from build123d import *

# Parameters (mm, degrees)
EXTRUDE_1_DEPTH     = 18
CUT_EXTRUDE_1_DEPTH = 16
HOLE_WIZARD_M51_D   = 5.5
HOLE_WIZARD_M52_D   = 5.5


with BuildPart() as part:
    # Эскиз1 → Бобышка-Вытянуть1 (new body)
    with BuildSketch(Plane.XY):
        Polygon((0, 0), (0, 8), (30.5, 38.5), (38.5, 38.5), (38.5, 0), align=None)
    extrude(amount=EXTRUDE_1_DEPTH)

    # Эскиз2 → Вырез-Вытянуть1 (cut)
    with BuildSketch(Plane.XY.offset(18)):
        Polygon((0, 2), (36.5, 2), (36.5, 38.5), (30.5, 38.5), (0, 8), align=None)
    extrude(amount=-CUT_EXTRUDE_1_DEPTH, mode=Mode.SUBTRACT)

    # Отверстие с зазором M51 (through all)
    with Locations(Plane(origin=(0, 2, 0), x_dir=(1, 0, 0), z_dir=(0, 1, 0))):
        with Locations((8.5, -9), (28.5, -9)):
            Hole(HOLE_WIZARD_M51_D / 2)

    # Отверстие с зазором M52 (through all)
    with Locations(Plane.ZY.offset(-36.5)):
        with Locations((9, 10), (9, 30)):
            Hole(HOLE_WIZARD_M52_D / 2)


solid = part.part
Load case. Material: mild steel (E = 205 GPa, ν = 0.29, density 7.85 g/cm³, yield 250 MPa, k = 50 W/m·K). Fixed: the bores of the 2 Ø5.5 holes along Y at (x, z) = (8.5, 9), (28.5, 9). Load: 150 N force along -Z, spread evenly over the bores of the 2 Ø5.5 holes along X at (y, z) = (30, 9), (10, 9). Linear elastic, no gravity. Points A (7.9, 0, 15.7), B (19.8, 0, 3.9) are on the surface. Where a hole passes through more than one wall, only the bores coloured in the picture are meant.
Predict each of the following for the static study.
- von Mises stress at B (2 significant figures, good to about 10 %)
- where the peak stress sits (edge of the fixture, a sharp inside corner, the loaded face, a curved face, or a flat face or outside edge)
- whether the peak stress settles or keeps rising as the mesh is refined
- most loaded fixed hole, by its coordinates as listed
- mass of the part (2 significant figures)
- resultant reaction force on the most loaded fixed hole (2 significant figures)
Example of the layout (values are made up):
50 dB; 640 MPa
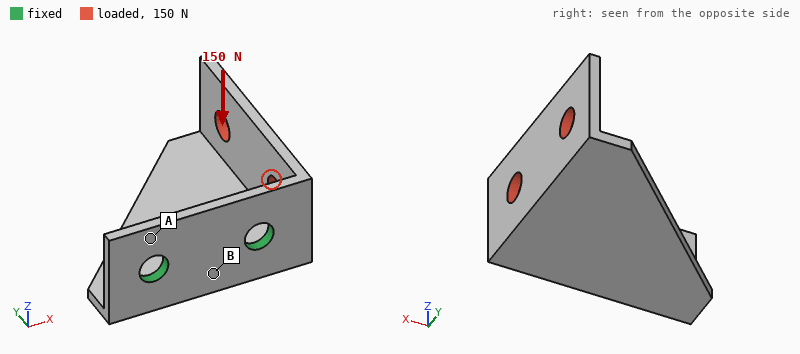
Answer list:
35 MPa; edge of the fixture; keeps rising; (28.5, 9); 33 g; 180 N
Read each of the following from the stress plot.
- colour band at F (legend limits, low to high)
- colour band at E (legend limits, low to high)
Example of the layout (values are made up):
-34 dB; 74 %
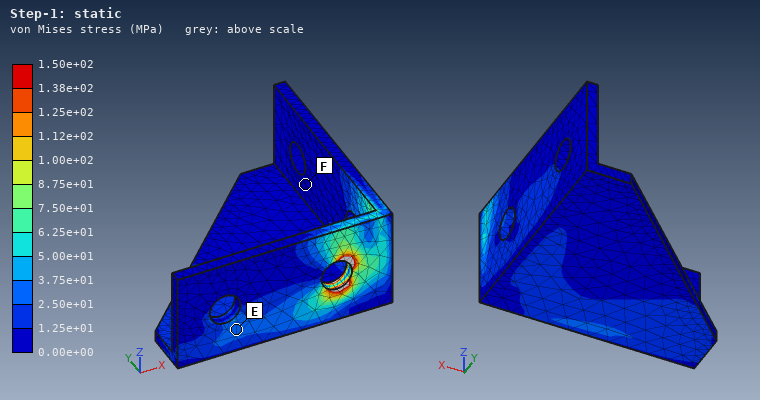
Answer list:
0.00e+00 to 1.25e+01 MPa; 2.50e+01 to 3.75e+01 MPa
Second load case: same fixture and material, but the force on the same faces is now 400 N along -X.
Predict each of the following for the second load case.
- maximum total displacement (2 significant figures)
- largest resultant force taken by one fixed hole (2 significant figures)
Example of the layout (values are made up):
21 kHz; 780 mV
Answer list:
0.16 mm; 390 N
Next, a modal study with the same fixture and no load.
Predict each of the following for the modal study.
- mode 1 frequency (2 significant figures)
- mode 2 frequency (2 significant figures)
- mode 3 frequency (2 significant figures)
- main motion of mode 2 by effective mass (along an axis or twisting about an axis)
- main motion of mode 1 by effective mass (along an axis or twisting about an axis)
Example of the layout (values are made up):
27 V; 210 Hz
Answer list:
1900 Hz; 3000 Hz; 6400 Hz; along X; along Z
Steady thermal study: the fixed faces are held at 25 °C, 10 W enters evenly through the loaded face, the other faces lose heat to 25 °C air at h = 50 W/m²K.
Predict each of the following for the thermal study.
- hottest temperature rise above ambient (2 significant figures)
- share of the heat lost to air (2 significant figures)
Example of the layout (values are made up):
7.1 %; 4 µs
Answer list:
56 K; 45 %
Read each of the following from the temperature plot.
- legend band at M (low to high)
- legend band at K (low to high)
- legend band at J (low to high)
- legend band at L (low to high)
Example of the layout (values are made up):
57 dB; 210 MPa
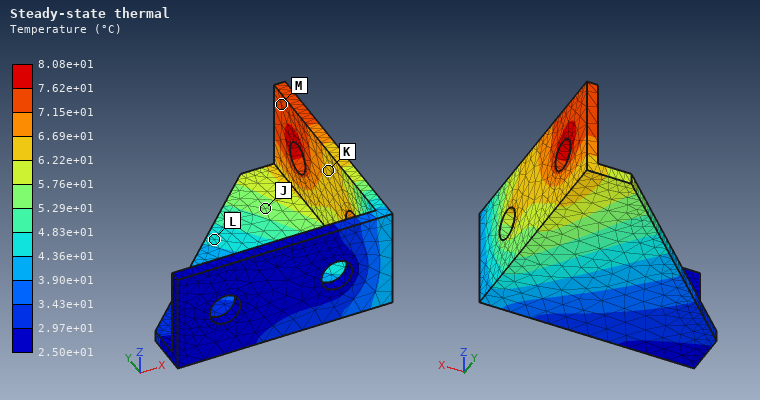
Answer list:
7.15e+01 to 7.62e+01 °C; 6.22e+01 to 6.69e+01 °C; 5.29e+01 to 5.76e+01 °C; 4.36e+01 to 4.83e+01 °C
